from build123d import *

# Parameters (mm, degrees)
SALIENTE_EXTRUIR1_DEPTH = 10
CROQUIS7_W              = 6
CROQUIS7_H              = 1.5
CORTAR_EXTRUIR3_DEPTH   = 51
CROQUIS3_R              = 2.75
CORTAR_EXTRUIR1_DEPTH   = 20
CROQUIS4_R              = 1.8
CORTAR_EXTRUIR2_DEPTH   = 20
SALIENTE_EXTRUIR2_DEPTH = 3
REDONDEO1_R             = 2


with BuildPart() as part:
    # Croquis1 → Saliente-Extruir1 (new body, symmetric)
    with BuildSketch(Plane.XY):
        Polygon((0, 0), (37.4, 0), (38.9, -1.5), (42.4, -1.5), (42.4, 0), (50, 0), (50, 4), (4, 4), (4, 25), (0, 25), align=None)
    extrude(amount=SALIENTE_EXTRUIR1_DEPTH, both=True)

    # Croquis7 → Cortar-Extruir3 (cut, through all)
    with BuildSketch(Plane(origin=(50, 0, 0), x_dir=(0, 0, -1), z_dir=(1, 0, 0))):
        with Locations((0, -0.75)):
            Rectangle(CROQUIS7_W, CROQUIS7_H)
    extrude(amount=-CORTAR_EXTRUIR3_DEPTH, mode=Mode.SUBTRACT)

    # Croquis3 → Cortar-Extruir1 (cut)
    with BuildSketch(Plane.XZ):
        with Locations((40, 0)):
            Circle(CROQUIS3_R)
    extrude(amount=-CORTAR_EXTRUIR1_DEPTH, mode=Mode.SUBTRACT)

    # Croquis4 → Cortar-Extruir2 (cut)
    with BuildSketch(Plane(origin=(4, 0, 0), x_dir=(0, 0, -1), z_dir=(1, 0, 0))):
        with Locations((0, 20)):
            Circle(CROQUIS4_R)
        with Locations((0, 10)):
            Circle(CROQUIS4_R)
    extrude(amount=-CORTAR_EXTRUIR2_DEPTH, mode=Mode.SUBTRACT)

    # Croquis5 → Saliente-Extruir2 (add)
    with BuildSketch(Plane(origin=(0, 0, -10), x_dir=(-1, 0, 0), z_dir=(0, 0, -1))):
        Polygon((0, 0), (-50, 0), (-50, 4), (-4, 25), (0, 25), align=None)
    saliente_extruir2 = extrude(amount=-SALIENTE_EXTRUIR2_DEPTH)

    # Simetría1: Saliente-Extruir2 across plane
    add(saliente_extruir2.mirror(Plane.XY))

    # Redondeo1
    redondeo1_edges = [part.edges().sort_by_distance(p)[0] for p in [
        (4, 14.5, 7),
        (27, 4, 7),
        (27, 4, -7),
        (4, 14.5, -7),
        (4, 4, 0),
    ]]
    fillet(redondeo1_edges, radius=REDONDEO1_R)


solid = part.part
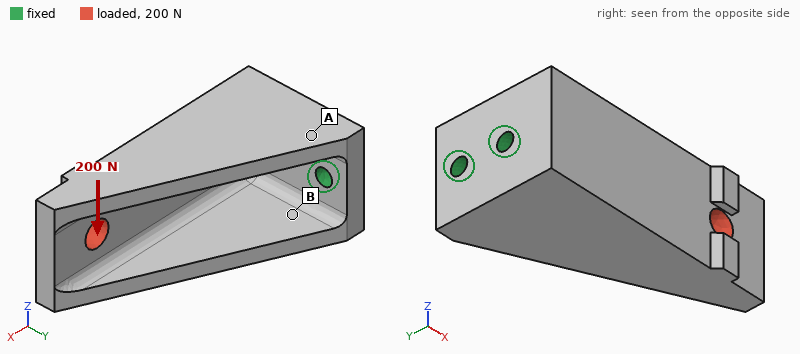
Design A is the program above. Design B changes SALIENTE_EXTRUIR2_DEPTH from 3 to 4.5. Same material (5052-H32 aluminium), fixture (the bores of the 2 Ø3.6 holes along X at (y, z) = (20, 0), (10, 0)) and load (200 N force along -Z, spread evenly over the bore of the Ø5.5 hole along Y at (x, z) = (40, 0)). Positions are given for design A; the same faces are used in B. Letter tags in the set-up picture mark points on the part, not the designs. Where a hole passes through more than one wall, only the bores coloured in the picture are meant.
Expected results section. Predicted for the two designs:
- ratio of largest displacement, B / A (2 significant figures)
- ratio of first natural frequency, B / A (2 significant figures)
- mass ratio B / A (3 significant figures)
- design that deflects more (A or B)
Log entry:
0.81
1.0
1.17
A
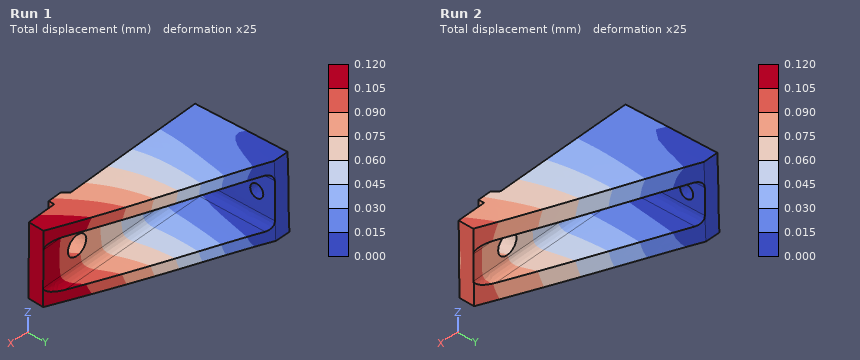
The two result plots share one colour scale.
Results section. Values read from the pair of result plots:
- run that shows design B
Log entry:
Run 2
